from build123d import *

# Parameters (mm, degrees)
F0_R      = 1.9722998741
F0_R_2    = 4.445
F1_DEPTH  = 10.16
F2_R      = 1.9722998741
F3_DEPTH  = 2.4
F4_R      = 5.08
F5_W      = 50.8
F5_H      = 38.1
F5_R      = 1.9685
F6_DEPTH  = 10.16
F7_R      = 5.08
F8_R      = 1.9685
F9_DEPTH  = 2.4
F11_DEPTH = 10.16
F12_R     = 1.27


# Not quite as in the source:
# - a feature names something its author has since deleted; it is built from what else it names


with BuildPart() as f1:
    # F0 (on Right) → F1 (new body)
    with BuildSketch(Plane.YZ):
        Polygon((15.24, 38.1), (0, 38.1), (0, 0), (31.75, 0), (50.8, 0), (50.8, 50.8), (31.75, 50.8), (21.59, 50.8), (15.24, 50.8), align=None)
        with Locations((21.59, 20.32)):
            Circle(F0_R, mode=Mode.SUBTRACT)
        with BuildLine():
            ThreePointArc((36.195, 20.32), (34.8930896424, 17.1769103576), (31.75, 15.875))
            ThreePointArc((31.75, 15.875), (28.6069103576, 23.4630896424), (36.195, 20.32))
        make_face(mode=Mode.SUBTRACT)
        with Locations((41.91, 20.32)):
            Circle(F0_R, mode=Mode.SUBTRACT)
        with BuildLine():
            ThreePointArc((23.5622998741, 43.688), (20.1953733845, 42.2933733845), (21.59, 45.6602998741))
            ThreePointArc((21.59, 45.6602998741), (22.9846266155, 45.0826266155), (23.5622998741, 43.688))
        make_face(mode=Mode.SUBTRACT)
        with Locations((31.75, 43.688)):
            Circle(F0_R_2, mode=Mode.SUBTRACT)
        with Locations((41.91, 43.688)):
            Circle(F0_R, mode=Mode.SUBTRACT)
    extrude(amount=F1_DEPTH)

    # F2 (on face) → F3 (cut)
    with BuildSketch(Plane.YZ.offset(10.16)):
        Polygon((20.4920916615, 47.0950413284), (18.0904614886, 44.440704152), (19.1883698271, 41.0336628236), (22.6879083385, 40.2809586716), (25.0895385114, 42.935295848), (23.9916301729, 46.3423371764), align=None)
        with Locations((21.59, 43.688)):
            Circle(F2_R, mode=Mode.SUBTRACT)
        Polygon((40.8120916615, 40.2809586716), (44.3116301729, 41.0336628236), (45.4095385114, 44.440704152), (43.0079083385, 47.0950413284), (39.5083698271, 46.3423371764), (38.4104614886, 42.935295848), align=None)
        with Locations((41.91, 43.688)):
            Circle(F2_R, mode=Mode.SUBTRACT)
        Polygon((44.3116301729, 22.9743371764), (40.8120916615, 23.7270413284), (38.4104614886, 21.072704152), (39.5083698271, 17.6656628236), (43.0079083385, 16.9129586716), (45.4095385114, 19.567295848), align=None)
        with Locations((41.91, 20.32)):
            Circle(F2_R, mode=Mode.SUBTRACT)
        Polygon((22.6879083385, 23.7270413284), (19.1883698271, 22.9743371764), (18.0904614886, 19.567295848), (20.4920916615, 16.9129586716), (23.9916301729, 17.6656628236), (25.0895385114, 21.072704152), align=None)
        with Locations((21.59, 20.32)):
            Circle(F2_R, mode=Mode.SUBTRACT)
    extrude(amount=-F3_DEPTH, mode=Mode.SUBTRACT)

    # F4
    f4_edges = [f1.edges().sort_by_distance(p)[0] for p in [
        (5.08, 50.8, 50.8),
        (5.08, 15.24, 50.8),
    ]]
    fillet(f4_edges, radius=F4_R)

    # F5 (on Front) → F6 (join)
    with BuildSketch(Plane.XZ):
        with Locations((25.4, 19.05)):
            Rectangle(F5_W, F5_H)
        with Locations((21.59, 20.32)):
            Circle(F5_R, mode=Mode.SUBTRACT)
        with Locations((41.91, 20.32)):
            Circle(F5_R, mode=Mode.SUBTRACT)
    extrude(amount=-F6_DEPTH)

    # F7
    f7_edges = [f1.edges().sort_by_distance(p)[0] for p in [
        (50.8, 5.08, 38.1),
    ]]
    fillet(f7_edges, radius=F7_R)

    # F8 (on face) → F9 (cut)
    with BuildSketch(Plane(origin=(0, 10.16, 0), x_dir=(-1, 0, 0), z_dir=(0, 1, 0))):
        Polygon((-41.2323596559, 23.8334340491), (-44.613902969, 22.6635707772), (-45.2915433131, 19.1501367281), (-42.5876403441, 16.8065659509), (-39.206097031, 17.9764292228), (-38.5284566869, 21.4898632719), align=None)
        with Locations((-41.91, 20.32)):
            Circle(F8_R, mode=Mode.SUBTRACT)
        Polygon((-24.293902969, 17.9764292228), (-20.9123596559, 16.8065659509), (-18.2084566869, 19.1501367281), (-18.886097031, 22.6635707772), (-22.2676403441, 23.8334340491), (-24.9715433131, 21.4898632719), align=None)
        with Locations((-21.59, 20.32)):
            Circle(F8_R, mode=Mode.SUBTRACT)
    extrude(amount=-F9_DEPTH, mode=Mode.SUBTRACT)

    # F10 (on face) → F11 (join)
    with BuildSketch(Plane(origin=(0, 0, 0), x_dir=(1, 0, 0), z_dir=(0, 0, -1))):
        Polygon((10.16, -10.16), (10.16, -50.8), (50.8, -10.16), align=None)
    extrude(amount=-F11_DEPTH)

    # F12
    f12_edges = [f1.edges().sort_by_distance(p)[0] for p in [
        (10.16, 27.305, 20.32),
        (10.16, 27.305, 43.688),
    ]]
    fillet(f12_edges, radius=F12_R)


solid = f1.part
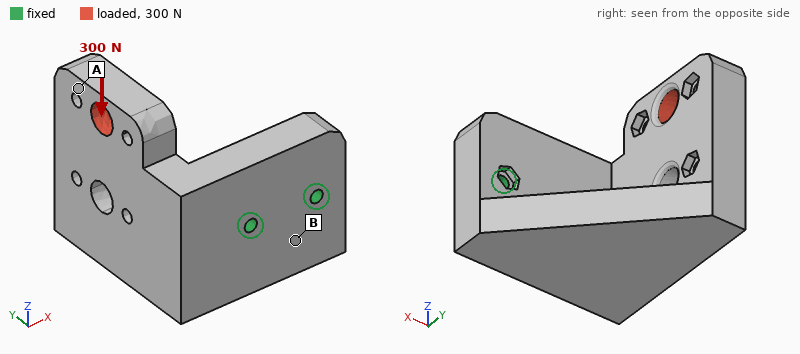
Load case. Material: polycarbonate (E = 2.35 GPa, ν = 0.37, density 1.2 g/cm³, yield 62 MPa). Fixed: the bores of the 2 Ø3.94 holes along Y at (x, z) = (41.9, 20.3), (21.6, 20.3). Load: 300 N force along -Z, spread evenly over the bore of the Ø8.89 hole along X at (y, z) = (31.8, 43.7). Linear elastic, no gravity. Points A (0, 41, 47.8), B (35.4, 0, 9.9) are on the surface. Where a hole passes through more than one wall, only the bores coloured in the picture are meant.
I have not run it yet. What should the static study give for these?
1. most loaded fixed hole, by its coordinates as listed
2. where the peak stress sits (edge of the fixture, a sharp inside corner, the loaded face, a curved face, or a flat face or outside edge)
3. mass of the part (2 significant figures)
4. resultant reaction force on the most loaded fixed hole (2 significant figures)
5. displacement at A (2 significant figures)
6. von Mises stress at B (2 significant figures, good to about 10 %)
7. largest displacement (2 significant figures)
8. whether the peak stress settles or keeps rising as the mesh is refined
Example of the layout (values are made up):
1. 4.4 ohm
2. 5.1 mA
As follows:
1. (21.6, 20.3)
2. edge of the fixture
3. 55 g
4. 510 N
5. 0.77 mm
6. 5.7 MPa
7. 0.90 mm
8. keeps rising
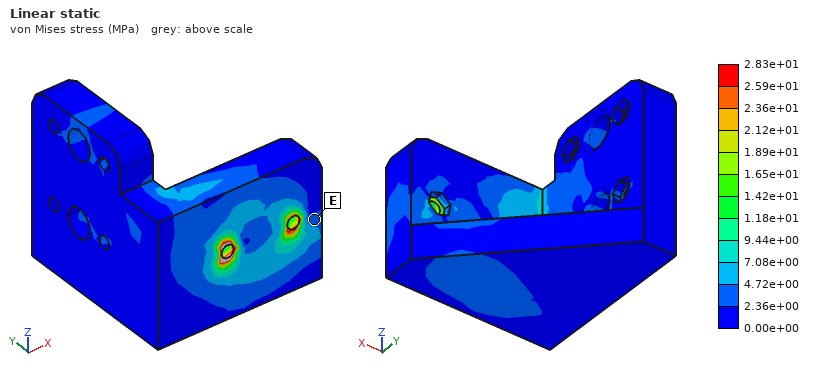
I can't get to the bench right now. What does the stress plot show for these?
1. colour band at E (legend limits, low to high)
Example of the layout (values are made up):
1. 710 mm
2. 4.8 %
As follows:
1. 2.36e+00 to 4.72e+00 MPa
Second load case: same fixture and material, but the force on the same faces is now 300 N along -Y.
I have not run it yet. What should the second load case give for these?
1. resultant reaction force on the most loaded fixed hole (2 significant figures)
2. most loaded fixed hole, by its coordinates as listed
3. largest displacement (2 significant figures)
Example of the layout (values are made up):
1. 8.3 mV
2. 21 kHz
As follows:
1. 460 N
2. (21.6, 20.3)
3. 0.83 mm
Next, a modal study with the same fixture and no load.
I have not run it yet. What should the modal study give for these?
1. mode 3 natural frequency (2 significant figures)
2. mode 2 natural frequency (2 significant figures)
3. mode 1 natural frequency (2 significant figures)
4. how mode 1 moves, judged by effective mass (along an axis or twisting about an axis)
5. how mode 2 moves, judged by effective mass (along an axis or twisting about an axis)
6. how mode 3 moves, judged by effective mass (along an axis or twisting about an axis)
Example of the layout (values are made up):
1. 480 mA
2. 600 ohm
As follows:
1. 1700 Hz
2. 880 Hz
3. 640 Hz
4. along Z
5. along X
6. along Y
